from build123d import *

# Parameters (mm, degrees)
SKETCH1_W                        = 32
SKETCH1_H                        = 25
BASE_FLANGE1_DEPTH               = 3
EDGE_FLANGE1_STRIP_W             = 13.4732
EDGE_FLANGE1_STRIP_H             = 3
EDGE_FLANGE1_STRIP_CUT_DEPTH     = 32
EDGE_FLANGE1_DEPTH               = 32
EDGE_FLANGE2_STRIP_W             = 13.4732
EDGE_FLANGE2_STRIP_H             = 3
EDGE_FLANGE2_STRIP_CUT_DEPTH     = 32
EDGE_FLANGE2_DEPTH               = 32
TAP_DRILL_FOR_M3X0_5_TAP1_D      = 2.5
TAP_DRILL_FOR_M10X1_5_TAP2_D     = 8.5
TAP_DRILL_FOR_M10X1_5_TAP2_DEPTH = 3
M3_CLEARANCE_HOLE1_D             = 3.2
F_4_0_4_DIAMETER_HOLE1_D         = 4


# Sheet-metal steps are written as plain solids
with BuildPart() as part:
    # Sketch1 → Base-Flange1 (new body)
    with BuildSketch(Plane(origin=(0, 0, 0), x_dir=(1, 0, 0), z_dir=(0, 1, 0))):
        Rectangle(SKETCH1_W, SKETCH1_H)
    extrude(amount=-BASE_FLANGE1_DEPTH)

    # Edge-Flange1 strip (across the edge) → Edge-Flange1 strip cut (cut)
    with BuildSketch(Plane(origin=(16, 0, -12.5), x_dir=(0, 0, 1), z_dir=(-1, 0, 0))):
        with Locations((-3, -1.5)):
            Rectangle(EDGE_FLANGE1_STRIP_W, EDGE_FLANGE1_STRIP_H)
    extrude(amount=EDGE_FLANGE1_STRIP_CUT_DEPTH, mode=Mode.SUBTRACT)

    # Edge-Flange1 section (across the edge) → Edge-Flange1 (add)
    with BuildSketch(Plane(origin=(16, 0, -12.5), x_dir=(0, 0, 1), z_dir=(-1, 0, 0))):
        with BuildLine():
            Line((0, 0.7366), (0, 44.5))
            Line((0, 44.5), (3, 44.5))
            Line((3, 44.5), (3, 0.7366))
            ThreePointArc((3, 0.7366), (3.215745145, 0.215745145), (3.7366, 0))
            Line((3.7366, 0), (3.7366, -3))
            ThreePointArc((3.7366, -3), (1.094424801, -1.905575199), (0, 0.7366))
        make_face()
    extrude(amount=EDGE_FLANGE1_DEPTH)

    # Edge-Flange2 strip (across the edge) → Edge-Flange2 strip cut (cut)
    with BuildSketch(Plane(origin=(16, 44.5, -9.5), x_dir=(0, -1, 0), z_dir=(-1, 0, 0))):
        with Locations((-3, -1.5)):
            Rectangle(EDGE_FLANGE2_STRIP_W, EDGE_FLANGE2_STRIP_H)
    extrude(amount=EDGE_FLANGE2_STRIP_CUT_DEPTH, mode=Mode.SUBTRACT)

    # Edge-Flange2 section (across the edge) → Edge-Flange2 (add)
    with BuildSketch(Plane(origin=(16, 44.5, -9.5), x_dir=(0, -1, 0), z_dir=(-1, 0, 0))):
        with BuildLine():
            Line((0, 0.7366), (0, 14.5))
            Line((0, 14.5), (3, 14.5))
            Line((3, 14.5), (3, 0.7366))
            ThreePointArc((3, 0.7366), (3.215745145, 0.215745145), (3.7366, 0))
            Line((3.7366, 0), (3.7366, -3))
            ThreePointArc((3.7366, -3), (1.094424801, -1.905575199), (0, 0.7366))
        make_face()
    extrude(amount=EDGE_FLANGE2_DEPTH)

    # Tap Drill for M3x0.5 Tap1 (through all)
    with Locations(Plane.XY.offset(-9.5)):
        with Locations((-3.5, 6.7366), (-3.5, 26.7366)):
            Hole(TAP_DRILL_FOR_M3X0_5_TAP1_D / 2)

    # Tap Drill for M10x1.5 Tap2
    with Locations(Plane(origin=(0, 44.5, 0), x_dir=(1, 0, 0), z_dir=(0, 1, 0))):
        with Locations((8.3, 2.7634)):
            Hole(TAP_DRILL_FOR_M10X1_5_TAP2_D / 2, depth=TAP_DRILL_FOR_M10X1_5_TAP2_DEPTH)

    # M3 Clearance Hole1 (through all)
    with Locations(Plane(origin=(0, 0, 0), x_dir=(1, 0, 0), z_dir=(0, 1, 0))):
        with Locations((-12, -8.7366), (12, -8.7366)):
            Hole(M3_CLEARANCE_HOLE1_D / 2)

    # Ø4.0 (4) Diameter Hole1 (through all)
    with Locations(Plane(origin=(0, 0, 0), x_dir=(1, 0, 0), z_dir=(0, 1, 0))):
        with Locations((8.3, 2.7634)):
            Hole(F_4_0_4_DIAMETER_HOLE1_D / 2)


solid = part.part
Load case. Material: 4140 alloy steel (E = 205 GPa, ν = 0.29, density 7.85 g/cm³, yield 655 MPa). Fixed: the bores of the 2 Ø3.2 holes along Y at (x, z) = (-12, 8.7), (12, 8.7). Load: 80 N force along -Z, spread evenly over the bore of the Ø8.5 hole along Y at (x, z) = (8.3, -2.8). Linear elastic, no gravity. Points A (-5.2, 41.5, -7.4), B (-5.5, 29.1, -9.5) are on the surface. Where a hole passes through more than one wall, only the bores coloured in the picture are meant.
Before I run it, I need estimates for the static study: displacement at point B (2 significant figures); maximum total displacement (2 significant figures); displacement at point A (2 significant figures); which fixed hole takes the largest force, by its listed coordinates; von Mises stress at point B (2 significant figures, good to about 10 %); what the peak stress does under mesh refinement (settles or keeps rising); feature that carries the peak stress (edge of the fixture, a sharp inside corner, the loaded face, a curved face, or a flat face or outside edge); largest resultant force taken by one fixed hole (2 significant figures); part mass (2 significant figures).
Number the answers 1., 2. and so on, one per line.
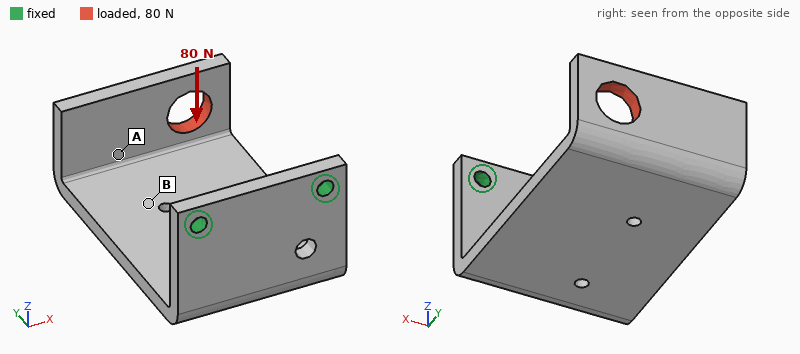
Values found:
1. 0.23 mm
2. 0.42 mm
3. 0.35 mm
4. (12, 8.7)
5. 27 MPa
6. keeps rising
7. edge of the fixture
8. 71 N
9. 60 g
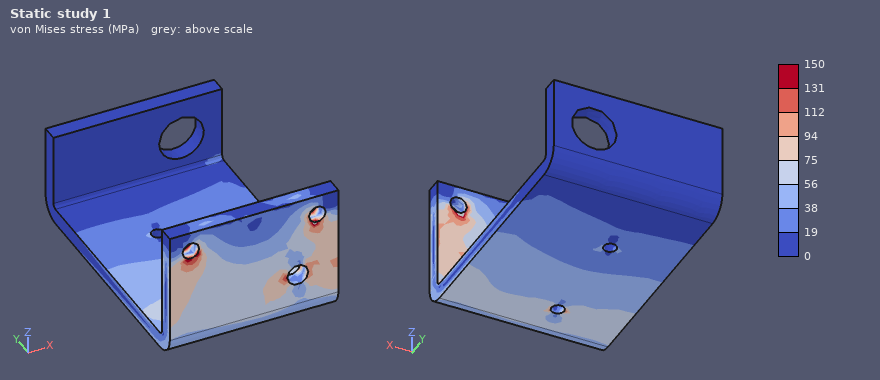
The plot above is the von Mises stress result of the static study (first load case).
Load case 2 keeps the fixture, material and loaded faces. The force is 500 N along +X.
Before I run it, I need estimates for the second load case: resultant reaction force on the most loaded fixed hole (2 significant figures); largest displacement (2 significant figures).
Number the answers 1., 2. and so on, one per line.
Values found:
1. 960 N
2. 0.70 mm
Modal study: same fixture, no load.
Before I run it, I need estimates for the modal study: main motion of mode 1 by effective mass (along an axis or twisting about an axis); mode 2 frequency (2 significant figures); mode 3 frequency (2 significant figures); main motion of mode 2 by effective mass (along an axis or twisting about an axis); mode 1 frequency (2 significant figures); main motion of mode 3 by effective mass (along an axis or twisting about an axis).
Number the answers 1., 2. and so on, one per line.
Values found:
1. along Z
2. 1100 Hz
3. 2000 Hz
4. along X
5. 520 Hz
6. along Y
